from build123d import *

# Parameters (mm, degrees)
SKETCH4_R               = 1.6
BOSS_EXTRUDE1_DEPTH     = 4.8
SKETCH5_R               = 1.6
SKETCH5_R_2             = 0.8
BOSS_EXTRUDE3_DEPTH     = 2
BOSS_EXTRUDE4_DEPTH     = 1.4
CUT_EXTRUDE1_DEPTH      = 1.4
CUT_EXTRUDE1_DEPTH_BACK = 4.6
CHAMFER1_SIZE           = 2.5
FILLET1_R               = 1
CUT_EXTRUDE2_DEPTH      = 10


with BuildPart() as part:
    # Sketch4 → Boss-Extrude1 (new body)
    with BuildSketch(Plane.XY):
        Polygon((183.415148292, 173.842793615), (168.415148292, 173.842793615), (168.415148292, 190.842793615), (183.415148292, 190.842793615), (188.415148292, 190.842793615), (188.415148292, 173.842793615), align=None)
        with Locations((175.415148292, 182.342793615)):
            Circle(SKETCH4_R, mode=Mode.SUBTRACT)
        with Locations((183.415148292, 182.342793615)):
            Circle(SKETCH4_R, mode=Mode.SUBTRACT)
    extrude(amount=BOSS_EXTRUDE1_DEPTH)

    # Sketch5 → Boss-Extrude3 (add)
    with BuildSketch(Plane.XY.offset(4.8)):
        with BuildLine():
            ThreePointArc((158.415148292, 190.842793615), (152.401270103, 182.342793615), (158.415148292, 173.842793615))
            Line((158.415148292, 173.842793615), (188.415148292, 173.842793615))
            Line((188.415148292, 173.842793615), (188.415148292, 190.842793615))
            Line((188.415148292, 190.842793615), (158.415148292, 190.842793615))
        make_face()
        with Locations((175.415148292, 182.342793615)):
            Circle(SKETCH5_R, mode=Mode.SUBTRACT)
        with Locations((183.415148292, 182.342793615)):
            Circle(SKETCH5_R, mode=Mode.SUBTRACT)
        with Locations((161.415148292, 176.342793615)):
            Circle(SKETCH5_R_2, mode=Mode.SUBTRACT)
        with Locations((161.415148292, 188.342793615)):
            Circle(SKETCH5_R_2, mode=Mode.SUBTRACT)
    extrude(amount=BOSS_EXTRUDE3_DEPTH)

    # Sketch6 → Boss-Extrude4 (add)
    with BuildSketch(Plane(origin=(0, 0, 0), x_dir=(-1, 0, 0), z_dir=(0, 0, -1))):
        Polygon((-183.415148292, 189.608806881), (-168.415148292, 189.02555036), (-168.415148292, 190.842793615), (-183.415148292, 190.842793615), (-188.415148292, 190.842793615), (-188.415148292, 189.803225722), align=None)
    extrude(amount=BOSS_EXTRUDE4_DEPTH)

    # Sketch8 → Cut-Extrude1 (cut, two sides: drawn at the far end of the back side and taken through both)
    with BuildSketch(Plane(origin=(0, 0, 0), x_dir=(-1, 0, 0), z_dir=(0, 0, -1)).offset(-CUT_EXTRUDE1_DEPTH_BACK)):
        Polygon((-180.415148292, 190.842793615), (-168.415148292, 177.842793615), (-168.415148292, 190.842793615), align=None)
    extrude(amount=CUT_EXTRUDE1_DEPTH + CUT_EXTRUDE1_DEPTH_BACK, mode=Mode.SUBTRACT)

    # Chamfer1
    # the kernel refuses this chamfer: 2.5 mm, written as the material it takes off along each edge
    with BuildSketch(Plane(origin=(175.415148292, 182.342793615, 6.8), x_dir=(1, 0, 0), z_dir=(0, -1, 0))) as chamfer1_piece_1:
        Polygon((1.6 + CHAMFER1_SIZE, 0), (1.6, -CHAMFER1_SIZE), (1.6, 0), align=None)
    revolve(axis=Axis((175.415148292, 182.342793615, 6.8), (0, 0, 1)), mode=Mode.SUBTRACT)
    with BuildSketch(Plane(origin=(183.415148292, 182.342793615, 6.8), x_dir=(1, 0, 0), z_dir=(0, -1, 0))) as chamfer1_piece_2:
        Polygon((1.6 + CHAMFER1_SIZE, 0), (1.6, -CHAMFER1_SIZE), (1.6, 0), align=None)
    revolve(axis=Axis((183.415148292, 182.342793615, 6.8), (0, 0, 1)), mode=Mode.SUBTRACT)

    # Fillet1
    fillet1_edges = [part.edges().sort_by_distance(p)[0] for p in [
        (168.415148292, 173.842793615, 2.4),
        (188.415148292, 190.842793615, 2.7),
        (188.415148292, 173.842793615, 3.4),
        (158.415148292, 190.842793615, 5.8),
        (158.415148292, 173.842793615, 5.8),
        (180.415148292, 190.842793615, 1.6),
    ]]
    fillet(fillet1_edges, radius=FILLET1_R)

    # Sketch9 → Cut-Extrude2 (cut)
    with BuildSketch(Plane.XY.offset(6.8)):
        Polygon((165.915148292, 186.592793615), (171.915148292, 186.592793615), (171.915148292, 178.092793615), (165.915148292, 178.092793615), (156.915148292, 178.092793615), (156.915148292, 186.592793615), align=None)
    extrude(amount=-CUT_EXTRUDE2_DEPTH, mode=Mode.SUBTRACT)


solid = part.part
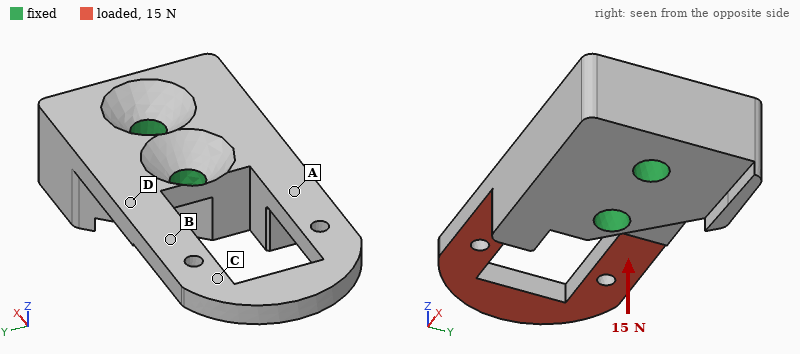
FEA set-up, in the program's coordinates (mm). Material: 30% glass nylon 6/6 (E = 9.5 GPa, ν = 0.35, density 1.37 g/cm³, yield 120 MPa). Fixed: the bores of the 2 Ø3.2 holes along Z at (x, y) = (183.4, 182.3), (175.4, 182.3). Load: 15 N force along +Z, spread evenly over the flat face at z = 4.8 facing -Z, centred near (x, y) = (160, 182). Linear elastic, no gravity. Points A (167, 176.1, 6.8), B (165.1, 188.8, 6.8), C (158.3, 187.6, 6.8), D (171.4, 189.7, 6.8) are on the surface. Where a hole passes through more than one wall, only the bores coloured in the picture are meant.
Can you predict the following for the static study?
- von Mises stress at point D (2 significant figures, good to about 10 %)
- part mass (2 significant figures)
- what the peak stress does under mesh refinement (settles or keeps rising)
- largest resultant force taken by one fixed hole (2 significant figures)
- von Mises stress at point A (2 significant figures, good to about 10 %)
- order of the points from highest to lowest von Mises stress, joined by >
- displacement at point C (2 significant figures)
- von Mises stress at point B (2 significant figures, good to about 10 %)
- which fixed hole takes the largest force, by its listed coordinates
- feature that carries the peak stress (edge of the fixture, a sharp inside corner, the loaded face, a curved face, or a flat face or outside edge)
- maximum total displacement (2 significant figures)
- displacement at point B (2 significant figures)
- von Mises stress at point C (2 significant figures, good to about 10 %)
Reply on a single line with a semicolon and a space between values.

16 MPa; 2.7 g; keeps rising; 35 N; 25 MPa; A > D > B > C; 0.27 mm; 9.0 MPa; (175.4, 182.3); a sharp inside corner; 0.38 mm; 0.14 mm; 3.2 MPa
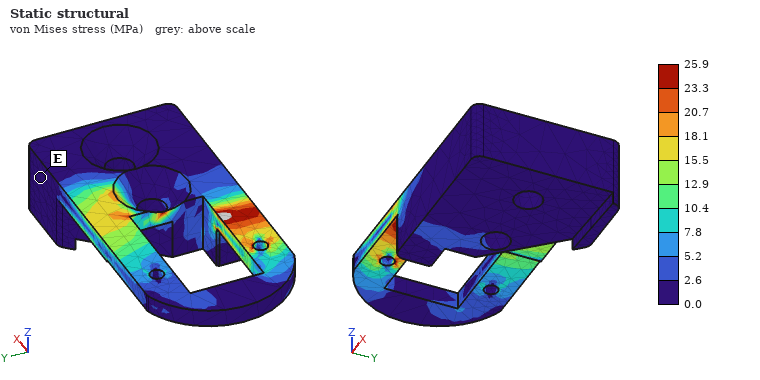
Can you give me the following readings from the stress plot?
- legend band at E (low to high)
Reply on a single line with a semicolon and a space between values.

0.0 to 2.6 MPa
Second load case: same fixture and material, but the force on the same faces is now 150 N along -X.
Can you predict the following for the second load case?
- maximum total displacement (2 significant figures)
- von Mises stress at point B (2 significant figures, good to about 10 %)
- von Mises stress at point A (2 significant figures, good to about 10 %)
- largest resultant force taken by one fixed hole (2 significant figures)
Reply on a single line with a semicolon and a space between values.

0.40 mm; 11 MPa; 20 MPa; 84 N
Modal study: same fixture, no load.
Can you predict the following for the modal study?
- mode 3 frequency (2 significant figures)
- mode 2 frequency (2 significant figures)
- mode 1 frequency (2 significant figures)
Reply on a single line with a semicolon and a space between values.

5400 Hz; 4800 Hz; 1900 Hz
